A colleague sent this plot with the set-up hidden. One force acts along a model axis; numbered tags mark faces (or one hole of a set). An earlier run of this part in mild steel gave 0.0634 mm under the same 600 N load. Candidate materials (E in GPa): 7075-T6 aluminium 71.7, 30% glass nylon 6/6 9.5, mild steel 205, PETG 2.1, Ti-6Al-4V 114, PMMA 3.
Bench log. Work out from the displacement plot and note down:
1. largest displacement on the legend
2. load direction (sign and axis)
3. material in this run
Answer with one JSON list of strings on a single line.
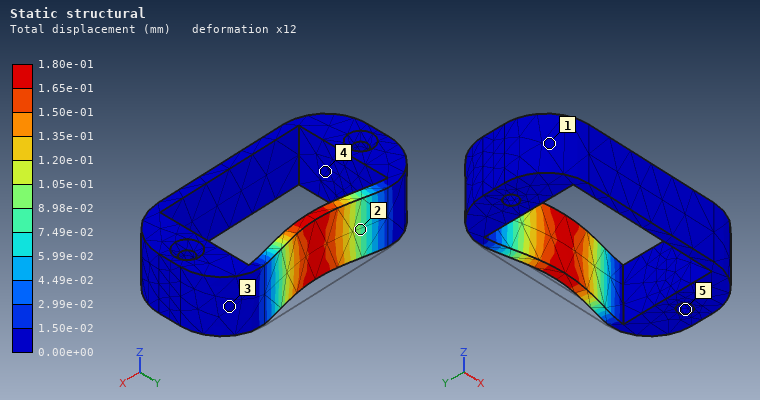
["1.80e-01 mm", "-Y", "7075-T6 aluminium"]
